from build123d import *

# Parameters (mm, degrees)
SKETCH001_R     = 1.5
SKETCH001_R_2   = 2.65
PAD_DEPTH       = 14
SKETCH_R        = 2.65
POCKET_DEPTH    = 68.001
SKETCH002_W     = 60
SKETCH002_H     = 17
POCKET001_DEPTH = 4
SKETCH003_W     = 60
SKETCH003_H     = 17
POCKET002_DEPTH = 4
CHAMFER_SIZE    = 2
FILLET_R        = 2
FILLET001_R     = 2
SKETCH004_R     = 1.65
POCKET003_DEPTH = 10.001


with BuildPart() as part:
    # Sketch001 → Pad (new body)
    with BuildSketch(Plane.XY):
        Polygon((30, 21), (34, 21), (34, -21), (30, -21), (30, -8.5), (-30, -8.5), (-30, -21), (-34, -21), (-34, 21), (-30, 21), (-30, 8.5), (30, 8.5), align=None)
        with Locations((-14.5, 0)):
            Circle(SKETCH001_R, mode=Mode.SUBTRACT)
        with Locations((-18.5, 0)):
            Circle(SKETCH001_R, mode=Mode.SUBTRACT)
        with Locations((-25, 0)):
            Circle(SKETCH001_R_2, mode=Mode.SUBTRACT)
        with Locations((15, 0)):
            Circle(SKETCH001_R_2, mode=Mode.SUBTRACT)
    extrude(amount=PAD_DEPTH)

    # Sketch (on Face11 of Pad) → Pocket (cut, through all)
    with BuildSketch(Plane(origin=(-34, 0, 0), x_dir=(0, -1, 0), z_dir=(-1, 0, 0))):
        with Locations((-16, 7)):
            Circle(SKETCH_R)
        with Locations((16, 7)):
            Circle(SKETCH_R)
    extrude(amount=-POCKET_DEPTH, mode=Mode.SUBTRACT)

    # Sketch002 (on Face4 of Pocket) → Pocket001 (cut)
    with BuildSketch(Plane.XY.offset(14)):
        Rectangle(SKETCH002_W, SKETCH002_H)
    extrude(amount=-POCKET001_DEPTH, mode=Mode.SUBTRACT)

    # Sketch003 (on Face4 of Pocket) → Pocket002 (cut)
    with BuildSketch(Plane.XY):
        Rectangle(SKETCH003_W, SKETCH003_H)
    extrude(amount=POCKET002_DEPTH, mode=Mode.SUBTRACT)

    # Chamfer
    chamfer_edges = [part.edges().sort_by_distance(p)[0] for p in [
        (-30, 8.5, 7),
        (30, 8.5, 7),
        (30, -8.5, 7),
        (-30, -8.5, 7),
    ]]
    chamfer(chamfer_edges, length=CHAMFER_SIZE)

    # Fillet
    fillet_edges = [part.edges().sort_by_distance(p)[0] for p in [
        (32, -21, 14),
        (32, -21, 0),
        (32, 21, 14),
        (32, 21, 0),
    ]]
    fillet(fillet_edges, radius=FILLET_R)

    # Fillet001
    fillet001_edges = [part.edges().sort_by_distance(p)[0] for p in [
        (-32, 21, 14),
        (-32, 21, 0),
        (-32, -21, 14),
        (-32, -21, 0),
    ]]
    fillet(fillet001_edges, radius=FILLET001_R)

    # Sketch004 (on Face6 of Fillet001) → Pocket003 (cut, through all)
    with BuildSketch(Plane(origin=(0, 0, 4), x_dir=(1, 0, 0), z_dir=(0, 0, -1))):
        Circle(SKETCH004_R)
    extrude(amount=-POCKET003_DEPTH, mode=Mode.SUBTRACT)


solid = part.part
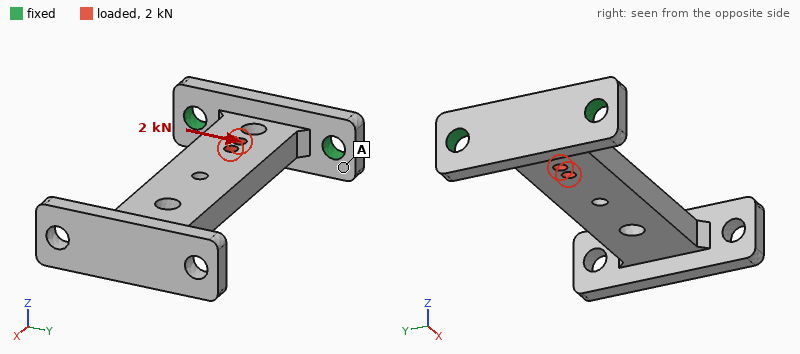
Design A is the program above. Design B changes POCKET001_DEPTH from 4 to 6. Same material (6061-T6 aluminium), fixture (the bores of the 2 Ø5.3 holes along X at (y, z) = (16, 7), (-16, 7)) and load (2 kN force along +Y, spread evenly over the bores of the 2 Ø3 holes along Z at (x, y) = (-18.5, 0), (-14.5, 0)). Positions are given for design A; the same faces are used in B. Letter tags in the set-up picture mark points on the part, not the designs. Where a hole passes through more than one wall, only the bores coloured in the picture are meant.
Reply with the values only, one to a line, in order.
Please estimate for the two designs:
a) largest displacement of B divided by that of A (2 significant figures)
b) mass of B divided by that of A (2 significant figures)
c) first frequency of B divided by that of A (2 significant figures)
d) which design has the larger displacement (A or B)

1.3
0.81
0.66
B
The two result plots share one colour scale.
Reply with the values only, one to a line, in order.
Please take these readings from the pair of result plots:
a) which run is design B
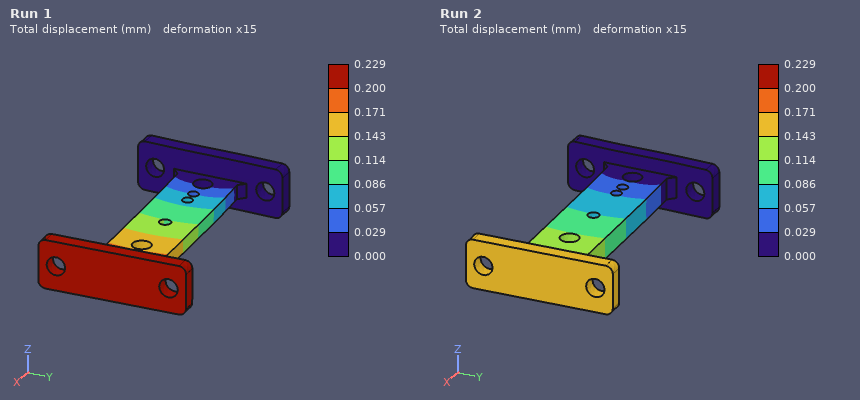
Run 1
